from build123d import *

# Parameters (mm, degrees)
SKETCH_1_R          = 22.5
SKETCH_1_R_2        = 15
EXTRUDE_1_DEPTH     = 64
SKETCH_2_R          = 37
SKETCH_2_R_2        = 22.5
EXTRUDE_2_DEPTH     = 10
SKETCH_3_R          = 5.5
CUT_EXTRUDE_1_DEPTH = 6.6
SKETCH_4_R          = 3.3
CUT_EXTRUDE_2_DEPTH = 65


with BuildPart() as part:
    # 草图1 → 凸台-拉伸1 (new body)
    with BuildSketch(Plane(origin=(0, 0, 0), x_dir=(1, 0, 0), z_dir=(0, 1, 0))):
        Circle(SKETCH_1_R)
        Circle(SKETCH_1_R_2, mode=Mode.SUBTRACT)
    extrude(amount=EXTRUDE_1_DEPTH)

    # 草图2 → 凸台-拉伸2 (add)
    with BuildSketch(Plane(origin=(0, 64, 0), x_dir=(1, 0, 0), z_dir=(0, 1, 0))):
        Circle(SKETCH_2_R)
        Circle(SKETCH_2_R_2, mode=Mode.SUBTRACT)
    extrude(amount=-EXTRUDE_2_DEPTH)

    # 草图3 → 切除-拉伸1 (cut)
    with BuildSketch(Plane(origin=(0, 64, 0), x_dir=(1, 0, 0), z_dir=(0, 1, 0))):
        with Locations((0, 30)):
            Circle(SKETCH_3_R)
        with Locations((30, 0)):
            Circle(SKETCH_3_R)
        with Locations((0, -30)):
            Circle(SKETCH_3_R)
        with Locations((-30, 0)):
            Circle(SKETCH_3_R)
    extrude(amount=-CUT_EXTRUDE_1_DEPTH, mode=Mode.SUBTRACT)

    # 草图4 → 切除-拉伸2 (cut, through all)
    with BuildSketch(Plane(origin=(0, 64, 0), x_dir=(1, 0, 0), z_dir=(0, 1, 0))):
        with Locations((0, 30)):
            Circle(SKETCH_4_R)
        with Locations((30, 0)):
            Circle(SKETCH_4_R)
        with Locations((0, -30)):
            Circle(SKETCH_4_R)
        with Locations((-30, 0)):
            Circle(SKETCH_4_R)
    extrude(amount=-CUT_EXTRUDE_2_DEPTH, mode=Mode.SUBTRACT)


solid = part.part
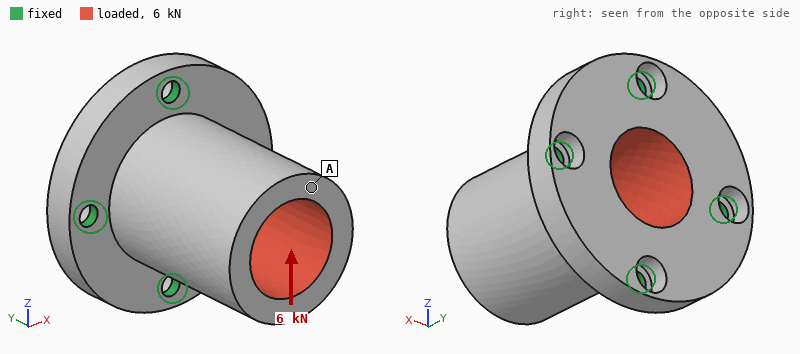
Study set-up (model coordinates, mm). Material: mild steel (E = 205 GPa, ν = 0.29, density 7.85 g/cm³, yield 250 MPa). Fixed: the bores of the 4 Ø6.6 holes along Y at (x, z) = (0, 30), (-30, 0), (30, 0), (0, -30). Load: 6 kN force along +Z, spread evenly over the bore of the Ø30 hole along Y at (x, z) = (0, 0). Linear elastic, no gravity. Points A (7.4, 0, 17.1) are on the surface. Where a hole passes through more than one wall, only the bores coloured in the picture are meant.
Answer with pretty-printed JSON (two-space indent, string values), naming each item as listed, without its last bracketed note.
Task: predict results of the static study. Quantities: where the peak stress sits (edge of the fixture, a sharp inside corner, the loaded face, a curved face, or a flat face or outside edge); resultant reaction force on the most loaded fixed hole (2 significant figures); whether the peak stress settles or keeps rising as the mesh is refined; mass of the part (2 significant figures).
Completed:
{
  "where the peak stress sits": "edge of the fixture",
  "resultant reaction force on the most loaded fixed hole": "2.7 kN",
  "whether the peak stress settles or keeps rising as the mesh is refined": "keeps rising",
  "mass of the part": "630 g"
}
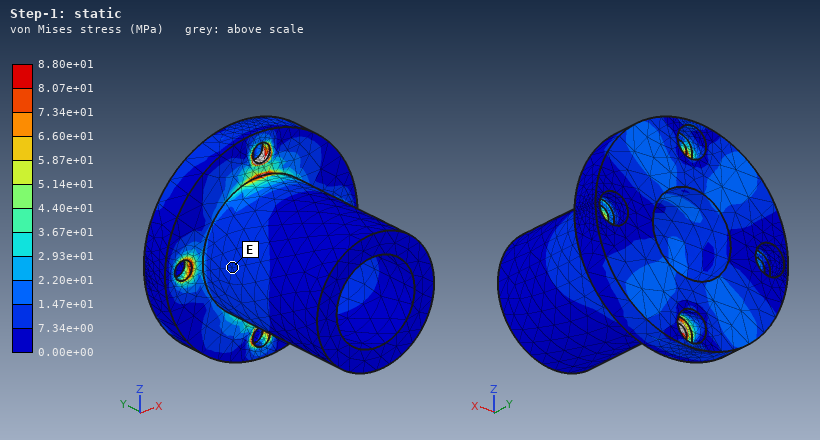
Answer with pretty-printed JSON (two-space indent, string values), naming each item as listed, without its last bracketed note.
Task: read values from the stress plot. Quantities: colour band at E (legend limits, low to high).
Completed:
{
  "colour band at E": "7.34e+00 to 1.47e+01 MPa"
}
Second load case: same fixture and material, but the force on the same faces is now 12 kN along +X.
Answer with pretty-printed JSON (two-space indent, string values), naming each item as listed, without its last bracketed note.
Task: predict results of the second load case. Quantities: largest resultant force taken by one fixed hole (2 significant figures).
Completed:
{
  "largest resultant force taken by one fixed hole": "5.4 kN"
}
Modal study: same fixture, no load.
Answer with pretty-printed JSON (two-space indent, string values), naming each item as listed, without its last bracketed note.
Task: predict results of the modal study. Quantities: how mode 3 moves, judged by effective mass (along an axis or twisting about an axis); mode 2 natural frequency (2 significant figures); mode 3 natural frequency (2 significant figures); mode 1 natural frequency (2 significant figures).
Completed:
{
  "how mode 3 moves, judged by effective mass": "along Y",
  "mode 2 natural frequency": "4800 Hz",
  "mode 3 natural frequency": "9200 Hz",
  "mode 1 natural frequency": "4800 Hz"
}
